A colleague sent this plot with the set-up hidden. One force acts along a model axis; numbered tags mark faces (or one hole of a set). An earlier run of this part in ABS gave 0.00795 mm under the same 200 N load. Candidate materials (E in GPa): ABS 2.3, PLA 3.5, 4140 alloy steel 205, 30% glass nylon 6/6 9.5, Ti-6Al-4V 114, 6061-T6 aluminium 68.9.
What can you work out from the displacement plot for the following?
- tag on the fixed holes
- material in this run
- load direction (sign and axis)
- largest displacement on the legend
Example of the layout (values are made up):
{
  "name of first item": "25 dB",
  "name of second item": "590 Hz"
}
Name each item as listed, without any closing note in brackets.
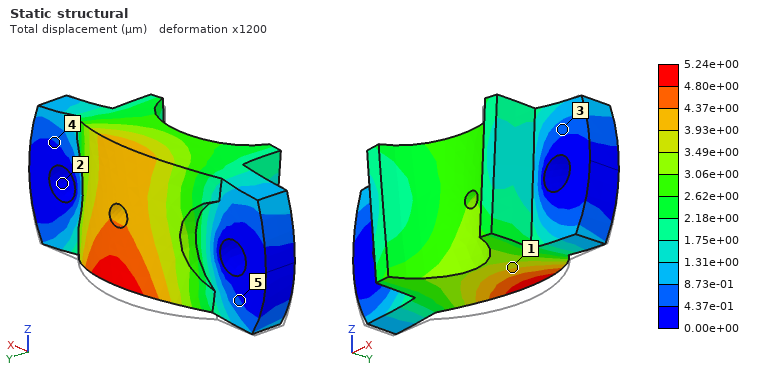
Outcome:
{
  "tag on the fixed holes": "2",
  "material in this run": "PLA",
  "load direction": "+Z",
  "largest displacement on the legend": "5.24e+00 µm"
}
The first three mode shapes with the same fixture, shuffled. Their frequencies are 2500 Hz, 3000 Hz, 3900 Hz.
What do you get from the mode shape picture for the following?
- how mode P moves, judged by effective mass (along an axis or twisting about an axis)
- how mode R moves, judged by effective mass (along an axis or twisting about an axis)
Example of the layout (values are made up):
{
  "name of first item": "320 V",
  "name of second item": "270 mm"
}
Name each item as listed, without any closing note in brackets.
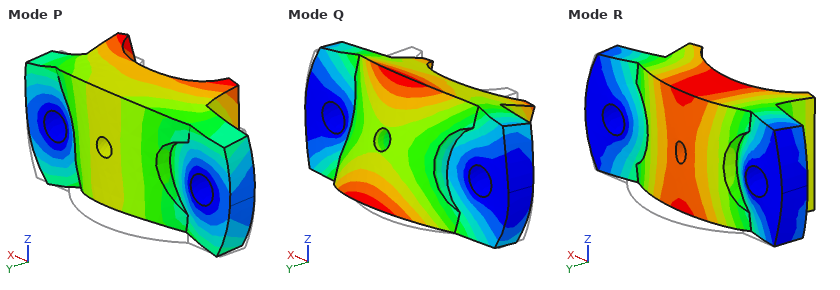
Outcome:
{
  "how mode P moves, judged by effective mass": "along Z",
  "how mode R moves, judged by effective mass": "along Y"
}
